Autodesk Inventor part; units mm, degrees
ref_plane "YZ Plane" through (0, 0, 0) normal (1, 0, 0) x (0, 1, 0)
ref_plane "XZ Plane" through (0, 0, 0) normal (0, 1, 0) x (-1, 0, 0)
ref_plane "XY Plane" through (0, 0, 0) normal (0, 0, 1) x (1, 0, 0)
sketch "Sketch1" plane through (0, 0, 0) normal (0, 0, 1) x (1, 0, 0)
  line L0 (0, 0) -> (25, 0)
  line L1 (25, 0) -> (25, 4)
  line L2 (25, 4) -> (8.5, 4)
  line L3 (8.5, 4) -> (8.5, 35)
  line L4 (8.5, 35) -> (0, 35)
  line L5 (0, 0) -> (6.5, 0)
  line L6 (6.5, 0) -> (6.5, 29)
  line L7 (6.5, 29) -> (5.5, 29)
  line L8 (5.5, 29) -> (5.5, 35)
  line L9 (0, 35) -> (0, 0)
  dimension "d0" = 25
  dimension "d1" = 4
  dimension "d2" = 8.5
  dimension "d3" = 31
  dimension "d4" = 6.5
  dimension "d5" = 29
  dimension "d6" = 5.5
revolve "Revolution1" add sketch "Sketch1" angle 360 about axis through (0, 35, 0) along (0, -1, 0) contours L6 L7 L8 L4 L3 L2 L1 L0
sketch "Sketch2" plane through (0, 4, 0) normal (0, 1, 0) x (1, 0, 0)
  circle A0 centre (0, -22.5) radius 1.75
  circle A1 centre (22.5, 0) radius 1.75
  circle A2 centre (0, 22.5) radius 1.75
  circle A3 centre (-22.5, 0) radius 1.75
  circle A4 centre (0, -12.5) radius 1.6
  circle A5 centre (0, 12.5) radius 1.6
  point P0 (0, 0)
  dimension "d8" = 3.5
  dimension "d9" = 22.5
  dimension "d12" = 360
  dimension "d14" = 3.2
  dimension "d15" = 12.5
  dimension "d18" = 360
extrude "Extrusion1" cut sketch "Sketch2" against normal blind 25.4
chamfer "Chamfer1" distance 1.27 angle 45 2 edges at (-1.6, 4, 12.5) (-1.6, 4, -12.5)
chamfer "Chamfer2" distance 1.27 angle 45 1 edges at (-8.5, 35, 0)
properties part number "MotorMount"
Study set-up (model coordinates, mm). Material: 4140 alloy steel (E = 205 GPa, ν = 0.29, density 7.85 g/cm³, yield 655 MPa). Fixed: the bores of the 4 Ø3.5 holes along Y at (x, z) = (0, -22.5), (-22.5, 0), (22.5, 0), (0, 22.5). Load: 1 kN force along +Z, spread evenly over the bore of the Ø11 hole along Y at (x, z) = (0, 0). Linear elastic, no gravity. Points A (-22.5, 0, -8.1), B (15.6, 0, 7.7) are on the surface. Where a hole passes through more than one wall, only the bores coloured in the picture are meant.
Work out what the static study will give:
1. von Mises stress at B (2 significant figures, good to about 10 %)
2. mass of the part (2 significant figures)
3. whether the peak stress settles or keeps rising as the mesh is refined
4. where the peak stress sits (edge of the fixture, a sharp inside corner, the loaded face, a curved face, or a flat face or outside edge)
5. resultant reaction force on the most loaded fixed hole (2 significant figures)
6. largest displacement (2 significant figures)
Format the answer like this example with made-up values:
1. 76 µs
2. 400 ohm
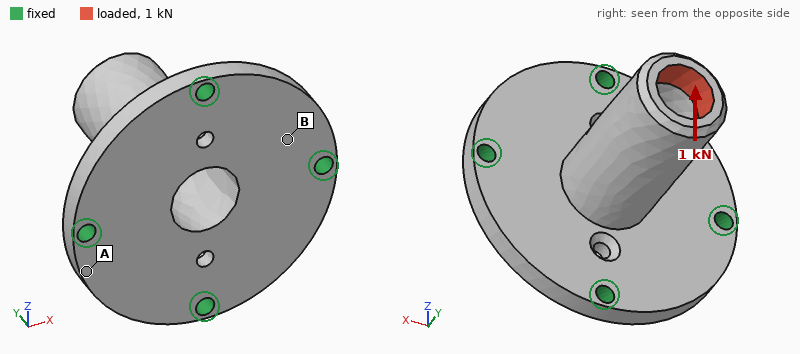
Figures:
1. 32 MPa
2. 80 g
3. keeps rising
4. edge of the fixture
5. 870 N
6. 79 µm
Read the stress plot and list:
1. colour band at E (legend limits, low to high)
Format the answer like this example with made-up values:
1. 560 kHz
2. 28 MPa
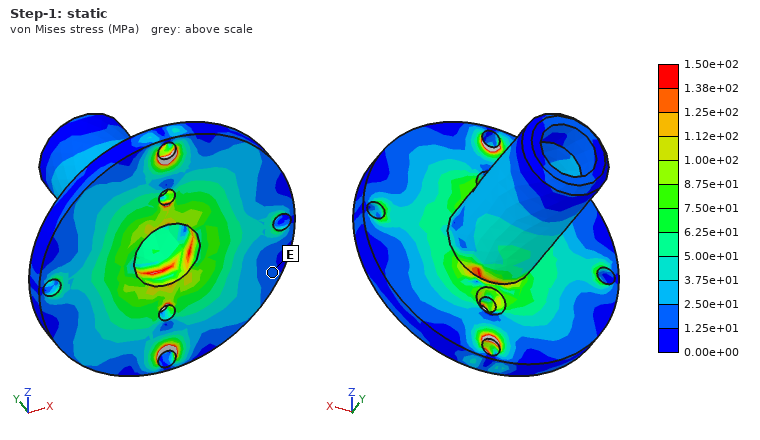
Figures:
1. 1.25e+01 to 2.50e+01 MPa
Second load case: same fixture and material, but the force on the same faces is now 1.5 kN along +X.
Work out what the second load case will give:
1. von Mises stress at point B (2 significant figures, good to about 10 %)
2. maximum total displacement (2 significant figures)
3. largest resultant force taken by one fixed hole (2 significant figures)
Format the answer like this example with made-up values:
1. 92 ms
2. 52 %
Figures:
1. 57 MPa
2. 0.12 mm
3. 1.3 kN
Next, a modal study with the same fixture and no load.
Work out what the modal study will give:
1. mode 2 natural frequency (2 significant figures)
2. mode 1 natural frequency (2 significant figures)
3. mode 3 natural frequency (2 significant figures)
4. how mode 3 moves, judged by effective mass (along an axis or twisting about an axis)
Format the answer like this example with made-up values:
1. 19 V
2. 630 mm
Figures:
1. 5700 Hz
2. 5600 Hz
3. 9800 Hz
4. along Y
